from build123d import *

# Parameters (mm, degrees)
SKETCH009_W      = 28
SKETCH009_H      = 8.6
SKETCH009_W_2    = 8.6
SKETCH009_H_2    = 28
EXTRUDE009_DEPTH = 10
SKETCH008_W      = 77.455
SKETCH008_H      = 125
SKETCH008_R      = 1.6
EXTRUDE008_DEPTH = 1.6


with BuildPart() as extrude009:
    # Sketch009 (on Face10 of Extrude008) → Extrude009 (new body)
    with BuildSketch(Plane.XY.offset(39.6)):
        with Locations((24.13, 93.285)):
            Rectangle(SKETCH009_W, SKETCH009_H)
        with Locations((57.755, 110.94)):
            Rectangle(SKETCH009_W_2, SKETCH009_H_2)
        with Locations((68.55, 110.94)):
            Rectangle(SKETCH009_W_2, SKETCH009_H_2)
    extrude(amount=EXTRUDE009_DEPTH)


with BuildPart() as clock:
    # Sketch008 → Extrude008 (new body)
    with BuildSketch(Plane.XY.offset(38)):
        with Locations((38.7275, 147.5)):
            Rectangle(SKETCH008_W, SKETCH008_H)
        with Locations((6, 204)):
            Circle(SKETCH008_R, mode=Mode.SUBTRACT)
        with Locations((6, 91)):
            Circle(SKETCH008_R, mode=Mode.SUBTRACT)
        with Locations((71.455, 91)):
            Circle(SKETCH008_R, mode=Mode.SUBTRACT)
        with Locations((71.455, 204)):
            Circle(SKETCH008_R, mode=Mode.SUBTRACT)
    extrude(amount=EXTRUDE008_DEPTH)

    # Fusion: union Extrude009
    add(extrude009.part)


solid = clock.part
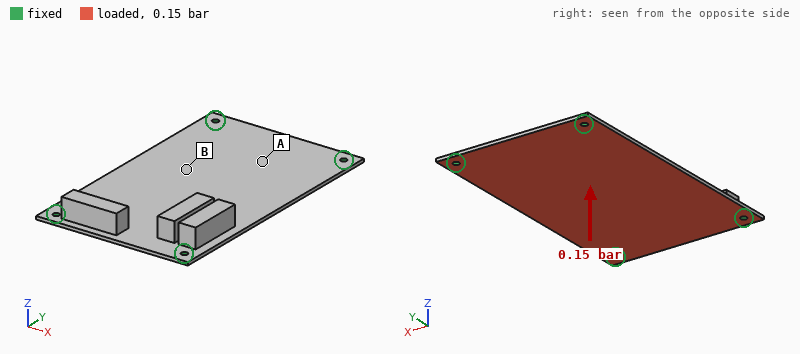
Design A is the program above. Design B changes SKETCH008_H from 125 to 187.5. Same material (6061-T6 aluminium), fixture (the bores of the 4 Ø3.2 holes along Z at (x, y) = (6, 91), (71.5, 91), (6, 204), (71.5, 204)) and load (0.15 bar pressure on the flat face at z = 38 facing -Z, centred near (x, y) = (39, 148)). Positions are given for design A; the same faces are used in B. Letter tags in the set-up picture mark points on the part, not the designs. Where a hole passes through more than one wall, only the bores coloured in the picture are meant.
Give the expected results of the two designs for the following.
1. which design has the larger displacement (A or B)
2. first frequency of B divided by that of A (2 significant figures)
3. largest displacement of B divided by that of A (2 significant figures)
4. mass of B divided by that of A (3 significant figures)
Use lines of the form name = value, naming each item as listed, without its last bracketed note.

which design has the larger displacement = A
first frequency of B divided by that of A = 0.99
largest displacement of B divided by that of A = 0.81
mass of B divided by that of A = 1.34
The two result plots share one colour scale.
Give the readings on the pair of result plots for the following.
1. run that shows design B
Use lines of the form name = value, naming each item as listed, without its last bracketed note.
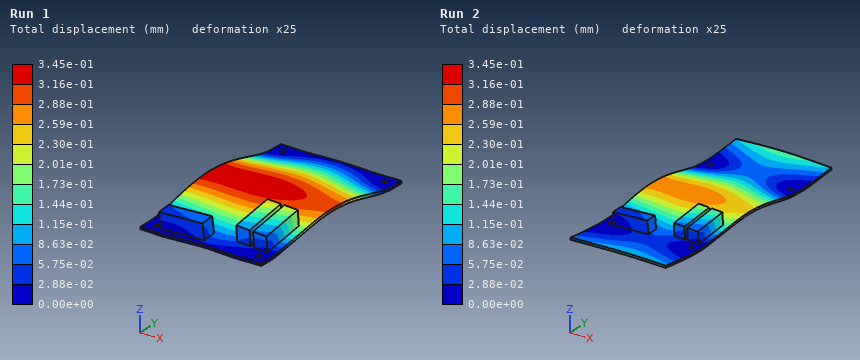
run that shows design B = Run 2
